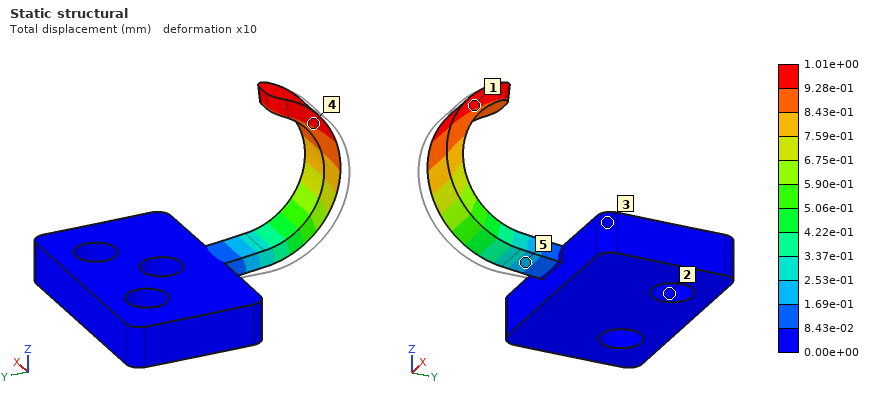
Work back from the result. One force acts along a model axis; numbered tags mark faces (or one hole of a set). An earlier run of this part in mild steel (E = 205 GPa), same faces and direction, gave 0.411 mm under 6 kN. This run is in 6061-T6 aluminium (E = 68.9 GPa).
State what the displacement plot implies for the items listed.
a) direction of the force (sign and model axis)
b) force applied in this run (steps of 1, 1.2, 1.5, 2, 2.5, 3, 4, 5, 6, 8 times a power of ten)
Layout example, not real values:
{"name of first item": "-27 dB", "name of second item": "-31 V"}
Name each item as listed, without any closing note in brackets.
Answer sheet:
{"direction of the force": "+Z", "force applied in this run": "5 kN"}
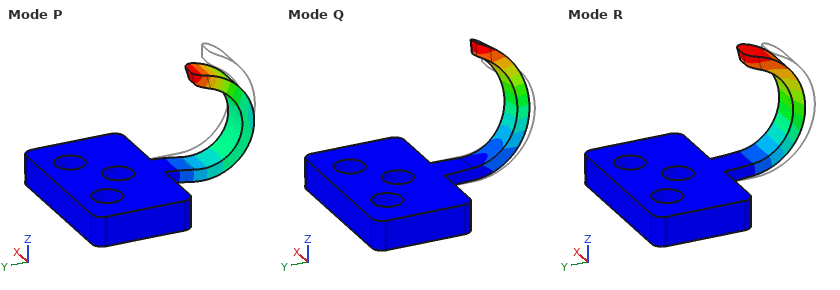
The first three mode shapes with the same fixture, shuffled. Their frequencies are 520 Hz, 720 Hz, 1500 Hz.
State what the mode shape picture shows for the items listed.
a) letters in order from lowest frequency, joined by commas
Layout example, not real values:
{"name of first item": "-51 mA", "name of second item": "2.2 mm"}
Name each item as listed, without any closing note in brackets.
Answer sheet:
{"letters in order from lowest frequency, joined by commas": "R, Q, P"}
